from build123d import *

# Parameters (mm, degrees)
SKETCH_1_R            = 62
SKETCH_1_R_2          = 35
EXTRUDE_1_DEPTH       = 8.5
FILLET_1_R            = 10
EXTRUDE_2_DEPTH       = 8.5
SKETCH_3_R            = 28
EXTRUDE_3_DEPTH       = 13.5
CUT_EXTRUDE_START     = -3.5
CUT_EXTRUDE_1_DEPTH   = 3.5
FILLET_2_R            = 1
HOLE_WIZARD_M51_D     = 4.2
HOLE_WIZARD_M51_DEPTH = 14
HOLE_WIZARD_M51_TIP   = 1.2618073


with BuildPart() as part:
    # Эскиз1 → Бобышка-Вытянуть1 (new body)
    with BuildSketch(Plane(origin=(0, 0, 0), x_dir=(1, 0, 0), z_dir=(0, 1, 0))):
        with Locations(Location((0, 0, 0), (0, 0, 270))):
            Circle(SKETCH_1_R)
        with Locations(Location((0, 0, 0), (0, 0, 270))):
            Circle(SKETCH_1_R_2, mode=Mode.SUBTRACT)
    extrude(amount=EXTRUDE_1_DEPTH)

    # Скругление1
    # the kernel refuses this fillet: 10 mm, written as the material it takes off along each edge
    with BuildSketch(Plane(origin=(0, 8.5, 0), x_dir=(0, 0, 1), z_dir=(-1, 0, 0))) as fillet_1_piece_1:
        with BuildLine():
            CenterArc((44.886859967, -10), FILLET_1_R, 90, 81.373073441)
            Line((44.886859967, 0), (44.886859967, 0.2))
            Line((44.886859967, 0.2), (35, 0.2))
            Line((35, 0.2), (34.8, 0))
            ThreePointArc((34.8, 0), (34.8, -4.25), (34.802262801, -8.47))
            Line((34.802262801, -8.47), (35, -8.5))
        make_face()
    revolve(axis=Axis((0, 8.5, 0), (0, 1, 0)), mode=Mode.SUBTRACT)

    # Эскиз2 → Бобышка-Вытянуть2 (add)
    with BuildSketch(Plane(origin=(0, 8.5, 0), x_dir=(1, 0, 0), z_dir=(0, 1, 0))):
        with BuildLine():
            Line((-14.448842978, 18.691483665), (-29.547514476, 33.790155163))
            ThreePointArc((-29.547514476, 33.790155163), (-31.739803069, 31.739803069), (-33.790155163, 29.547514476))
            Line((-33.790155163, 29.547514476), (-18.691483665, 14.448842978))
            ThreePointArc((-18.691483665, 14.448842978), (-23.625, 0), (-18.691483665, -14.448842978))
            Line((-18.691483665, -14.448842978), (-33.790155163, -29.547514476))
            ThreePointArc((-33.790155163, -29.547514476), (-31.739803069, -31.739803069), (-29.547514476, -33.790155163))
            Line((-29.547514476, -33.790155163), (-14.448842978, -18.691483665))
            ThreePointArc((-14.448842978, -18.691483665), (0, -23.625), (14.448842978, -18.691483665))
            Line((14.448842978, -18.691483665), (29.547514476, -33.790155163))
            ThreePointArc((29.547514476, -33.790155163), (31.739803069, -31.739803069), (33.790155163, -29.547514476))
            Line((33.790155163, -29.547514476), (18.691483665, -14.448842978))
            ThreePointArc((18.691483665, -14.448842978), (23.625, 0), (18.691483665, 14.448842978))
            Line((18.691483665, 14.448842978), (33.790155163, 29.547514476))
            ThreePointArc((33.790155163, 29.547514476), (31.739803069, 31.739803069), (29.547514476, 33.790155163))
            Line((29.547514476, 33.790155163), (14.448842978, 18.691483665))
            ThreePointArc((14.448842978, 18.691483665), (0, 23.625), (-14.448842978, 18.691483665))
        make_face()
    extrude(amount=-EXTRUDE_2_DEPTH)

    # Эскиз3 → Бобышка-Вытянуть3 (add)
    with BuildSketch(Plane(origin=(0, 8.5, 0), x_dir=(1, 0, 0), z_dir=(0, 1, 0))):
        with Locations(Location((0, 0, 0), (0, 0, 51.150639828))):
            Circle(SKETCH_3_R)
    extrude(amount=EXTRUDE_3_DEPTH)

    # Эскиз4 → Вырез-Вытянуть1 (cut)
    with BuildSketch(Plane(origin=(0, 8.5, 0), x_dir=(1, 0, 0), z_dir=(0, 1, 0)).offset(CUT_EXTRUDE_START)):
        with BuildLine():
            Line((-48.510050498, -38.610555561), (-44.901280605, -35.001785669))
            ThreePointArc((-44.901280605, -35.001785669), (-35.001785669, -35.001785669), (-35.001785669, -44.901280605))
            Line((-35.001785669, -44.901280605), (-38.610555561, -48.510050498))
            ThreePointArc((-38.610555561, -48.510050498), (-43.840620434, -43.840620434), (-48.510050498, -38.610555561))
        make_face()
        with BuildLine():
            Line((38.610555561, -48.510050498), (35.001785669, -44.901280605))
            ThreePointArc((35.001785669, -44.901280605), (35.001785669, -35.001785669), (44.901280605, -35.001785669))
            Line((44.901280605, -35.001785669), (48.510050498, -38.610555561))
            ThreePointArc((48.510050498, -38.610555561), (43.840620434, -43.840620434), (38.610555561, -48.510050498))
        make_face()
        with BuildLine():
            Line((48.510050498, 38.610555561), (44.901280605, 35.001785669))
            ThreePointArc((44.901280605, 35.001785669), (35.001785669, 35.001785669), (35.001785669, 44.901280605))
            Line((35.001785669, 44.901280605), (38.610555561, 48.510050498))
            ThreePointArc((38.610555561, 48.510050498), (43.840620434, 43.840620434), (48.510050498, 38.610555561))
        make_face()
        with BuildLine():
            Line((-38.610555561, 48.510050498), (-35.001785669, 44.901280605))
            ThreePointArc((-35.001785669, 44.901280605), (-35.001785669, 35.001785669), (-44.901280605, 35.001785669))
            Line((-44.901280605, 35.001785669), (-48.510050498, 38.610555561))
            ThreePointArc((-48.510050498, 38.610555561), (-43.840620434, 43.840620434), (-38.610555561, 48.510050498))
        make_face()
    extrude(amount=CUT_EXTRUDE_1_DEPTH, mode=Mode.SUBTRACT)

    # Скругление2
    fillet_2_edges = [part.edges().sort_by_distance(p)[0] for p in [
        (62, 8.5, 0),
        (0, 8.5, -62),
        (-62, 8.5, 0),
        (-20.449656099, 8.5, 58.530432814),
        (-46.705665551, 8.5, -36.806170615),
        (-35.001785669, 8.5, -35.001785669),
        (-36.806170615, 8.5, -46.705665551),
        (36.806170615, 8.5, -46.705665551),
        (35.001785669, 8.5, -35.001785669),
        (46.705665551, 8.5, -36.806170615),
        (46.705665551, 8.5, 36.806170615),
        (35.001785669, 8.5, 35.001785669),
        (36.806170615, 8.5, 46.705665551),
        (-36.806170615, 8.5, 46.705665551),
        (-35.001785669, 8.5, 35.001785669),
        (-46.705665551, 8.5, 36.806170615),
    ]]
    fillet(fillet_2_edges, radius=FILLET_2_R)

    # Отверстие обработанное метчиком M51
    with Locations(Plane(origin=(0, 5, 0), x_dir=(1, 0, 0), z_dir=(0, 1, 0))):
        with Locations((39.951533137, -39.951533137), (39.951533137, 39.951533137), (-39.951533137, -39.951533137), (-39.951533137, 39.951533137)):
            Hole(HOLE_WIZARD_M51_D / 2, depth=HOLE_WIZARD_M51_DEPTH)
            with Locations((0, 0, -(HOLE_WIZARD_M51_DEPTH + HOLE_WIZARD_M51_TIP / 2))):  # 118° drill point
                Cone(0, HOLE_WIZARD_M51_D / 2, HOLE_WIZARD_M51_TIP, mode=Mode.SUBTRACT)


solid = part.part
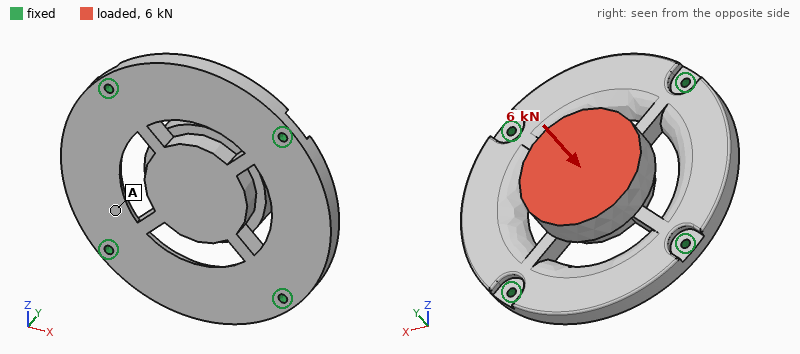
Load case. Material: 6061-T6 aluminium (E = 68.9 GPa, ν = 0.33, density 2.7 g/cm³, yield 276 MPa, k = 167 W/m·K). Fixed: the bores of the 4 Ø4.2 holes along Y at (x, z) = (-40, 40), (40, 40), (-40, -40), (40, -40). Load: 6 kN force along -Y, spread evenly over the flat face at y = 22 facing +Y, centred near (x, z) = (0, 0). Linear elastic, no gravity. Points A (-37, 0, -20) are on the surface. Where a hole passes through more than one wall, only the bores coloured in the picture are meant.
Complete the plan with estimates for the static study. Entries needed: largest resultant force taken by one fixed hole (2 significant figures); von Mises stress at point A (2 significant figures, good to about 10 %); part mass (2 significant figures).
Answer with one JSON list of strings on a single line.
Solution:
["2.5 kN", "30 MPa", "310 g"]
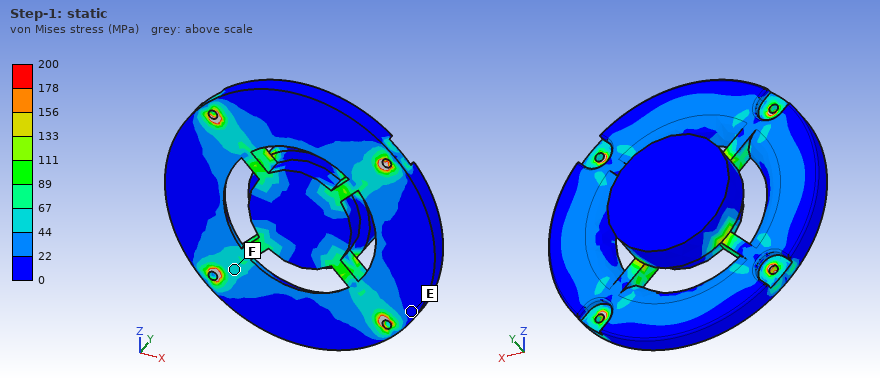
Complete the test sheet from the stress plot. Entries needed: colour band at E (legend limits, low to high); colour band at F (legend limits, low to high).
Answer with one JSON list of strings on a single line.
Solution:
["0 to 22 MPa", "44 to 67 MPa"]
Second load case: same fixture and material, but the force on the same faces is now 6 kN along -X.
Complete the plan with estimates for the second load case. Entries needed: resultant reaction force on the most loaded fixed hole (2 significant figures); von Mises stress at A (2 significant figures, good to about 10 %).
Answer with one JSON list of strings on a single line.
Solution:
["2.1 kN", "16 MPa"]
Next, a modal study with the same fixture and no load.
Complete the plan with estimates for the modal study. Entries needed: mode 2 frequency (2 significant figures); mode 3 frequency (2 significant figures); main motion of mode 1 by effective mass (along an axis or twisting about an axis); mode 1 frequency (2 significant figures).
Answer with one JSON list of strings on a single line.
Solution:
["3600 Hz", "4100 Hz", "along Y", "2600 Hz"]
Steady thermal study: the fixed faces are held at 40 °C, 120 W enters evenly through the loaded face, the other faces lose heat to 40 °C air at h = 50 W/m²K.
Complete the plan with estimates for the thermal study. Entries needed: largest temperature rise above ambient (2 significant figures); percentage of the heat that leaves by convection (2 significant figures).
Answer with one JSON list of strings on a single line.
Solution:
["66 K", "25 %"]
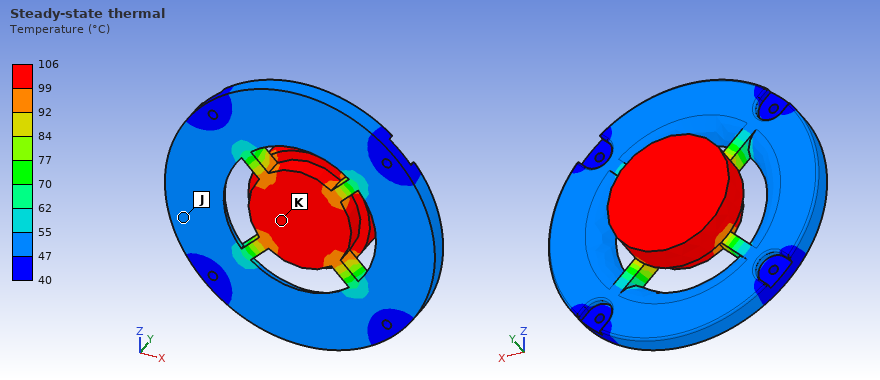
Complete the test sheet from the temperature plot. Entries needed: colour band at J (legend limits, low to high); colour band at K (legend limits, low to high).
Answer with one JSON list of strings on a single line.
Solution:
["47 to 55 °C", "99 to 106 °C"]
